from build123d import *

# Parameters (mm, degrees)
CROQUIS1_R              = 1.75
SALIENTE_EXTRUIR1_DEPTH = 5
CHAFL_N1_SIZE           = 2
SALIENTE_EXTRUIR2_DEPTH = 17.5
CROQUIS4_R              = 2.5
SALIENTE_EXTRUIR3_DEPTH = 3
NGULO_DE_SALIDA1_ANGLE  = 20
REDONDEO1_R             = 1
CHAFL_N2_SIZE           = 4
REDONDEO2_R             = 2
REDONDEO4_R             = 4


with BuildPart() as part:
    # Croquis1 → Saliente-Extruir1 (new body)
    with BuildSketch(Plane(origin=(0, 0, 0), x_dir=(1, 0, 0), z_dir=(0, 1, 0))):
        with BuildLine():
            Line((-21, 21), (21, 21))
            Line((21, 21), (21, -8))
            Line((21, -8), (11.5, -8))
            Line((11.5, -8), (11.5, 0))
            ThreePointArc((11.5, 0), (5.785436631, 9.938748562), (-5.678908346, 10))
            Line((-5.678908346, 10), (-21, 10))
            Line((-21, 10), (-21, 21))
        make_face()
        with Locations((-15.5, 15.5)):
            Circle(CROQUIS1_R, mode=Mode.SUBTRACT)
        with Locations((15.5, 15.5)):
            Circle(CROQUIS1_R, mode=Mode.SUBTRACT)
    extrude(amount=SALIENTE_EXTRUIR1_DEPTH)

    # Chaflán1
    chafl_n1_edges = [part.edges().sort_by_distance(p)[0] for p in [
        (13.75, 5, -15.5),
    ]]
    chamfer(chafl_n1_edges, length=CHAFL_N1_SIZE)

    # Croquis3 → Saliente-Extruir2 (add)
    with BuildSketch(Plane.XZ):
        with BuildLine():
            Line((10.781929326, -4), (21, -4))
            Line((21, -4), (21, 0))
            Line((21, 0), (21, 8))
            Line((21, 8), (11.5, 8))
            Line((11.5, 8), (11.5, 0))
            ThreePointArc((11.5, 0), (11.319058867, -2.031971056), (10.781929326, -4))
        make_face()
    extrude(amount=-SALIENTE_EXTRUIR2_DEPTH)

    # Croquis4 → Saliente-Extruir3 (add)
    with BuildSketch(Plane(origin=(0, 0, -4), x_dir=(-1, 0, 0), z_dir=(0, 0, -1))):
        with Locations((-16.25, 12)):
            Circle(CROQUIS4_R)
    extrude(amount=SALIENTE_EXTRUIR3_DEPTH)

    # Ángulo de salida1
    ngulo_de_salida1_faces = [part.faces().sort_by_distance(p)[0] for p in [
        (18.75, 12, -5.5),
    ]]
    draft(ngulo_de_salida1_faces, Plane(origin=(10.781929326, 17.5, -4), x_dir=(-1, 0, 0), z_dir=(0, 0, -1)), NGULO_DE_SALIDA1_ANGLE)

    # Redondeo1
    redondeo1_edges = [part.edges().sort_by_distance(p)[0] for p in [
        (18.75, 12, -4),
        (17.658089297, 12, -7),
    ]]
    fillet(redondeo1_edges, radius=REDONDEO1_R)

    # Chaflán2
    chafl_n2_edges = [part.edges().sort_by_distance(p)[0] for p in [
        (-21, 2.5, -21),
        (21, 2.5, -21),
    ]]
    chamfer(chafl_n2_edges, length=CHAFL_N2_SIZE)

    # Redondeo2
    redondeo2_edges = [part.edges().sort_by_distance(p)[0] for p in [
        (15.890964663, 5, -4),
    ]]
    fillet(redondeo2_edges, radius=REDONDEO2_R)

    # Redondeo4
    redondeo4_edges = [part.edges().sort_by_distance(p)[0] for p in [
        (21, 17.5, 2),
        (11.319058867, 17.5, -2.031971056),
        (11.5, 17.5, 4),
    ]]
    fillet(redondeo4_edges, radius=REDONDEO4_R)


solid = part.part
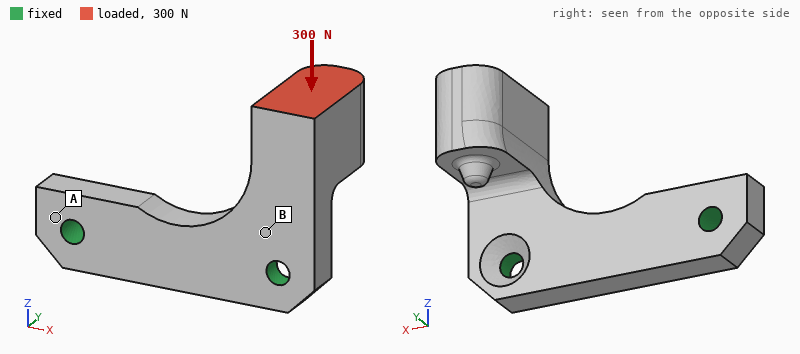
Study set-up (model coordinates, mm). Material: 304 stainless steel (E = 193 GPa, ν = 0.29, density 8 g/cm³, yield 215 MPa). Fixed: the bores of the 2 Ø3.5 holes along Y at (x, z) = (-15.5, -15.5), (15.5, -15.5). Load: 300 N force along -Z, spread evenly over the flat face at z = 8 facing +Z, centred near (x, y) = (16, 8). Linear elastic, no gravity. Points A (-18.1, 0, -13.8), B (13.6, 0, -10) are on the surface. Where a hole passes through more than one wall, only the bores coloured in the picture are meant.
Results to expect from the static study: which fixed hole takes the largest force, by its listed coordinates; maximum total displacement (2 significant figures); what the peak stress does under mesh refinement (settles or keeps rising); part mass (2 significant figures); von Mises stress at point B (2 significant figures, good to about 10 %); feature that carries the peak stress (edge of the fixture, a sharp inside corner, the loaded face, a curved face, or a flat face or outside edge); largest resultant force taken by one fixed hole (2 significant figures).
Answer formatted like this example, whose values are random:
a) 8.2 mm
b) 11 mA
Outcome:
a) (15.5, -15.5)
b) 28 µm
c) keeps rising
d) 35 g
e) 28 MPa
f) edge of the fixture
g) 300 N
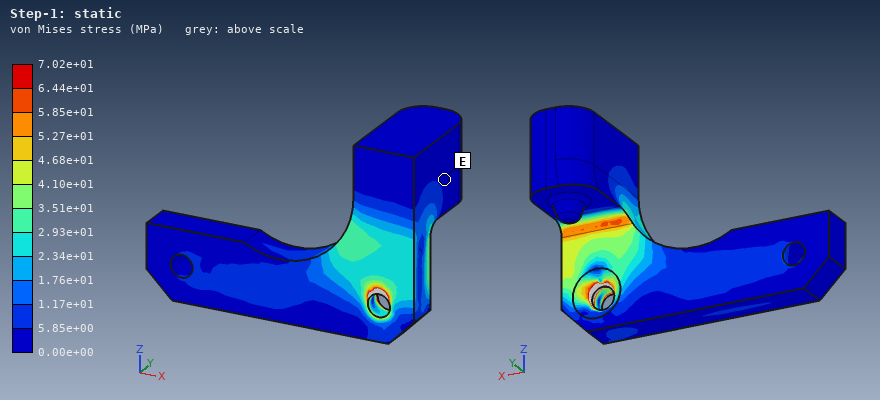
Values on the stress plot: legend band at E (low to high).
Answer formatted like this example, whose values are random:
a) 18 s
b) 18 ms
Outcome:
a) 0.00e+00 to 5.85e+00 MPa
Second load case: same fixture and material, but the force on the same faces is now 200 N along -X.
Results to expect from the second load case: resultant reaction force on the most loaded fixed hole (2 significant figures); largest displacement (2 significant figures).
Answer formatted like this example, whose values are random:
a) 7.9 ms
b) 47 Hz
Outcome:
a) 170 N
b) 16 µm
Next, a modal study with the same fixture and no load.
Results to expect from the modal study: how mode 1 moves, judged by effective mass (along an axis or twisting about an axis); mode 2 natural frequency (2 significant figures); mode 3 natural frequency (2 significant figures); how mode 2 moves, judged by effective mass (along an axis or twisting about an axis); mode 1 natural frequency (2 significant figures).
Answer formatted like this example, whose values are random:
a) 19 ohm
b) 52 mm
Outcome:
a) along Y
b) 6100 Hz
c) 13 kHz
d) along X
e) 3300 Hz
